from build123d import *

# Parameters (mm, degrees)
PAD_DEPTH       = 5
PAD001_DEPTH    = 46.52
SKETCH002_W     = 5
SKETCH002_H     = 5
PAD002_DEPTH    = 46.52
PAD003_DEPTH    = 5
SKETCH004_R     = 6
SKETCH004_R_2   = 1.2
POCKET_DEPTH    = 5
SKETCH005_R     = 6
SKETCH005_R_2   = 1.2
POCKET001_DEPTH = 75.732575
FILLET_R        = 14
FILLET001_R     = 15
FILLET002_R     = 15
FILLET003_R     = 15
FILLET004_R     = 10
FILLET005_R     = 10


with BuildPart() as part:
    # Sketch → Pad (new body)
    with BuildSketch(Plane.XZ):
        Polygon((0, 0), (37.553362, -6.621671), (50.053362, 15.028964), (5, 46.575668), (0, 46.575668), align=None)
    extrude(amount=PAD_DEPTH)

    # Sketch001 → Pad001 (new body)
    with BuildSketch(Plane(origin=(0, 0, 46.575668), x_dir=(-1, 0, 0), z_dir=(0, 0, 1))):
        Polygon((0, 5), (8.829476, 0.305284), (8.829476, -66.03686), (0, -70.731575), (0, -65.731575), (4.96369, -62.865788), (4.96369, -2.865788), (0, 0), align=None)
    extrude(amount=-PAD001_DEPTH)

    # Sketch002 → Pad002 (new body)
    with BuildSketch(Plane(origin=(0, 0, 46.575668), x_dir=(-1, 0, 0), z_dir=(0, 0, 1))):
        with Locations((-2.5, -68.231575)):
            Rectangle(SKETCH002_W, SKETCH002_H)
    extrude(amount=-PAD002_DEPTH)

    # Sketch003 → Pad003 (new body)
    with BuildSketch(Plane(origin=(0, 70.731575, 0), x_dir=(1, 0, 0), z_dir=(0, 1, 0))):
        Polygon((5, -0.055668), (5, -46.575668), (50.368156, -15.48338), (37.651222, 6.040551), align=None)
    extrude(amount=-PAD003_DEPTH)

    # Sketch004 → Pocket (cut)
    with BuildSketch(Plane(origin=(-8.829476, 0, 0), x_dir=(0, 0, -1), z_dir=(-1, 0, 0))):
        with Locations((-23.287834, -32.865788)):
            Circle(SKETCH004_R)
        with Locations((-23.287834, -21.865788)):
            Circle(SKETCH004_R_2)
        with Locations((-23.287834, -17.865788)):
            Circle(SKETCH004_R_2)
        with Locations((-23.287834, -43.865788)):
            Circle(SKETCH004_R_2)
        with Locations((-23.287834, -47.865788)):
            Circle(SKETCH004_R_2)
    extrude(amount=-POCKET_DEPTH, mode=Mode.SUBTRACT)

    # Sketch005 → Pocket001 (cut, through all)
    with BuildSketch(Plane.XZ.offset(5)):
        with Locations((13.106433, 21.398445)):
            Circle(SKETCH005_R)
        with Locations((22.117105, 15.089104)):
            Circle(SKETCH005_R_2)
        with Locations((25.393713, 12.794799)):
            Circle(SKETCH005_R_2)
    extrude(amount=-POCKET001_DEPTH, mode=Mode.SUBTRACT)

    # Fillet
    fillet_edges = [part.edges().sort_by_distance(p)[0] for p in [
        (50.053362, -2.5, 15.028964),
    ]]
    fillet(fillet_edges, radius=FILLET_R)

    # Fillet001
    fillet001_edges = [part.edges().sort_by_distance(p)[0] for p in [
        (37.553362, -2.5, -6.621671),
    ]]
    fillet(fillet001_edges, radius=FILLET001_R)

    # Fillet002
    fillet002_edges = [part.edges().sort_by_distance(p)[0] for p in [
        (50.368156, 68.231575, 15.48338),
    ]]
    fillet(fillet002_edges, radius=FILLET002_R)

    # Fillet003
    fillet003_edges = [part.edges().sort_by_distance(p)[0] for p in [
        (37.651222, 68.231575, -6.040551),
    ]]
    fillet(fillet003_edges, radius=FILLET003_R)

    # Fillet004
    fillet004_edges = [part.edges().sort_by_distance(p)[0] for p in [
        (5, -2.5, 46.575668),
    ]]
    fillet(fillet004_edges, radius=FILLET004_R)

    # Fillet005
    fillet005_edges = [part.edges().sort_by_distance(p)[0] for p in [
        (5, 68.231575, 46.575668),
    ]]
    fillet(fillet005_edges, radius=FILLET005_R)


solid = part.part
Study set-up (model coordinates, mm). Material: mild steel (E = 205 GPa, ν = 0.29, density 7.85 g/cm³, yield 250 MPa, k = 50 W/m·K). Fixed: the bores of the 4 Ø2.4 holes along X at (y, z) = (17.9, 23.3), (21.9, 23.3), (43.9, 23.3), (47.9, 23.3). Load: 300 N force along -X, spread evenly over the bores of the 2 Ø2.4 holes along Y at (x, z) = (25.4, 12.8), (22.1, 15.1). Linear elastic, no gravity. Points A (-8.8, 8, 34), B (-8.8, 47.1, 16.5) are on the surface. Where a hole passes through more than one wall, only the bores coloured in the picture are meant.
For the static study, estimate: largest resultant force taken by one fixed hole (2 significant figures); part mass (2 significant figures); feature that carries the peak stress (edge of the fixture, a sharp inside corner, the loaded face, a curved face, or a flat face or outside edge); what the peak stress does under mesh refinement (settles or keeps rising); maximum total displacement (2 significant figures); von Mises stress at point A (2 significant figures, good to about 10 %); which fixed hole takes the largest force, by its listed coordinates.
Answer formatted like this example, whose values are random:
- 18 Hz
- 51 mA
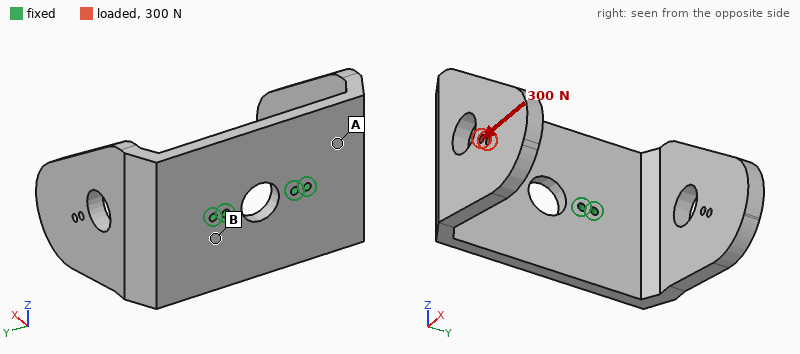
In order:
- 630 N
- 230 g
- edge of the fixture
- keeps rising
- 0.11 mm
- 32 MPa
- (17.9, 23.3)
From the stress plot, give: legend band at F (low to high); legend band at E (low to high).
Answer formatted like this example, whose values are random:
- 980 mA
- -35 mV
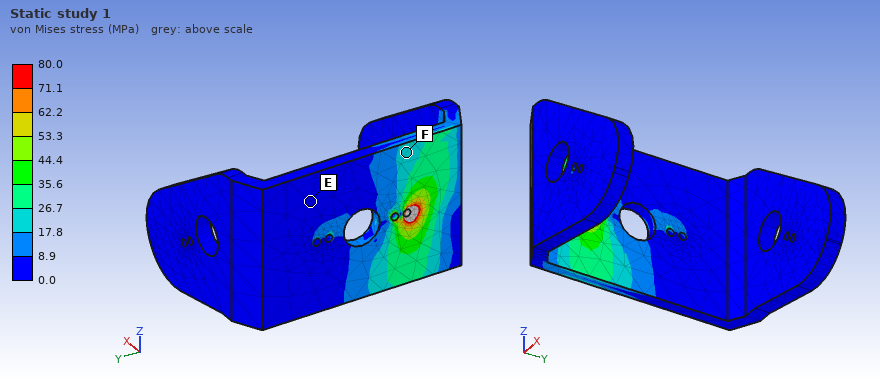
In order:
- 17.8 to 26.7 MPa
- 0.0 to 8.9 MPa
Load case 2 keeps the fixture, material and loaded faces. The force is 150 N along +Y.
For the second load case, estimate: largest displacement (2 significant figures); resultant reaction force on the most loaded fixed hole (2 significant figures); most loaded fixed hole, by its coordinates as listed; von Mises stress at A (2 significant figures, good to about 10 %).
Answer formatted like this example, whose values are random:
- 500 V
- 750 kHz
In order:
- 0.15 mm
- 310 N
- (17.9, 23.3)
- 33 MPa
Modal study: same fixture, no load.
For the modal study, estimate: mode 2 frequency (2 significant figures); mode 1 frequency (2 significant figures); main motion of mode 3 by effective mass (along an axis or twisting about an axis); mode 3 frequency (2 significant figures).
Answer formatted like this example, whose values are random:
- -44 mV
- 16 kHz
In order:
- 860 Hz
- 830 Hz
- along Z
- 1100 Hz
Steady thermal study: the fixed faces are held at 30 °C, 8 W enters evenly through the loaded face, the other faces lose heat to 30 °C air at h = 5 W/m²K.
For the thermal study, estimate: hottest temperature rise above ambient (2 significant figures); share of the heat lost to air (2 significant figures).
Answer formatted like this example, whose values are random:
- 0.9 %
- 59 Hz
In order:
- 57 K
- 13 %
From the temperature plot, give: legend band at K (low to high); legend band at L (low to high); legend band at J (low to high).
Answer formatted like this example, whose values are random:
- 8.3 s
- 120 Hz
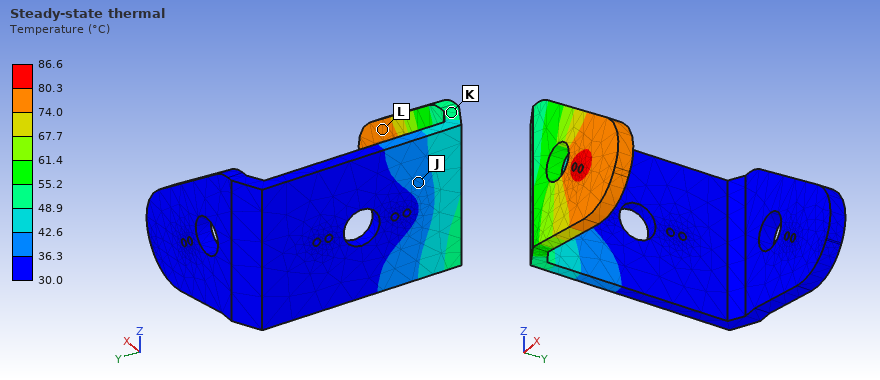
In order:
- 48.9 to 55.2 °C
- 74.0 to 80.3 °C
- 36.3 to 42.6 °C
